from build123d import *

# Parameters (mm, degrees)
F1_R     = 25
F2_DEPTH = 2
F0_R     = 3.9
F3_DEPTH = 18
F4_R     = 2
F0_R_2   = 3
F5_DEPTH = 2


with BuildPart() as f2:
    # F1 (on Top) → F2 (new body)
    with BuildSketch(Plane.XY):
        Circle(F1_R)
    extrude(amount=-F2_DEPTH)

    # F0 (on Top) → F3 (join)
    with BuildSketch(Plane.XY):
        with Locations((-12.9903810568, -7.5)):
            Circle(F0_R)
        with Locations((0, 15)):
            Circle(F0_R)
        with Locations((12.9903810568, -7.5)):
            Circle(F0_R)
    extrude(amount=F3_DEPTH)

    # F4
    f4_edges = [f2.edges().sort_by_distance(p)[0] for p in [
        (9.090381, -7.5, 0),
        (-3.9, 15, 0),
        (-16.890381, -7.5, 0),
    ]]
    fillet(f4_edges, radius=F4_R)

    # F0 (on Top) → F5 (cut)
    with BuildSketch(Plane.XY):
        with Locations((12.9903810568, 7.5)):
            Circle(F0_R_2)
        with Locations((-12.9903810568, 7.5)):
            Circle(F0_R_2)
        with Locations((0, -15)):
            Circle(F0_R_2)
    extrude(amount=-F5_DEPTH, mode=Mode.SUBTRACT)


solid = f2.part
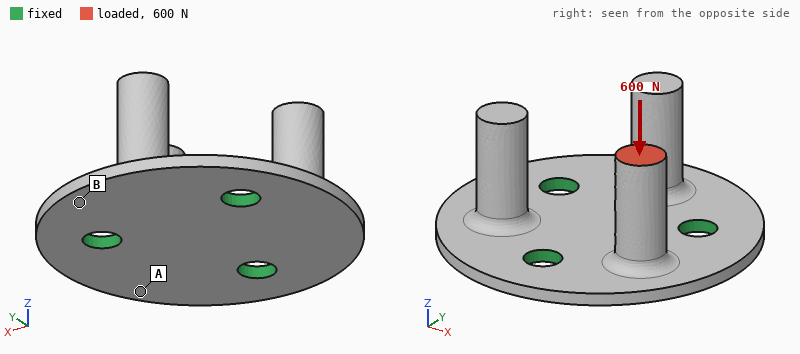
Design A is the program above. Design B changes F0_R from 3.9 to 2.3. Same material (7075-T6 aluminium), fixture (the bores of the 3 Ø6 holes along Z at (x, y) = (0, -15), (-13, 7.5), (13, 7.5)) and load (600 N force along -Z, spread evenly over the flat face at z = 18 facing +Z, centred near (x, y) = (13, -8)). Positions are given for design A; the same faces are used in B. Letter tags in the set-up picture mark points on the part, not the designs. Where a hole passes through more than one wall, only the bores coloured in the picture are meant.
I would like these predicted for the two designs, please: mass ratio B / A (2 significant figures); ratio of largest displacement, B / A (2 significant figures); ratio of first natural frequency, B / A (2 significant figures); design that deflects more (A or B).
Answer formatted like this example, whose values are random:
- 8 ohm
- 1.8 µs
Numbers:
- 0.73
- 1.1
- 1.3
- B
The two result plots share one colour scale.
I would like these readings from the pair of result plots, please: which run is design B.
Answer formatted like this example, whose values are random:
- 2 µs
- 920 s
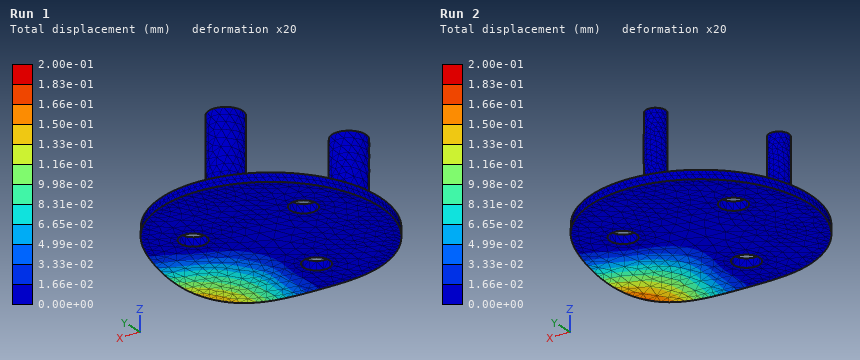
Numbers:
- Run 2
